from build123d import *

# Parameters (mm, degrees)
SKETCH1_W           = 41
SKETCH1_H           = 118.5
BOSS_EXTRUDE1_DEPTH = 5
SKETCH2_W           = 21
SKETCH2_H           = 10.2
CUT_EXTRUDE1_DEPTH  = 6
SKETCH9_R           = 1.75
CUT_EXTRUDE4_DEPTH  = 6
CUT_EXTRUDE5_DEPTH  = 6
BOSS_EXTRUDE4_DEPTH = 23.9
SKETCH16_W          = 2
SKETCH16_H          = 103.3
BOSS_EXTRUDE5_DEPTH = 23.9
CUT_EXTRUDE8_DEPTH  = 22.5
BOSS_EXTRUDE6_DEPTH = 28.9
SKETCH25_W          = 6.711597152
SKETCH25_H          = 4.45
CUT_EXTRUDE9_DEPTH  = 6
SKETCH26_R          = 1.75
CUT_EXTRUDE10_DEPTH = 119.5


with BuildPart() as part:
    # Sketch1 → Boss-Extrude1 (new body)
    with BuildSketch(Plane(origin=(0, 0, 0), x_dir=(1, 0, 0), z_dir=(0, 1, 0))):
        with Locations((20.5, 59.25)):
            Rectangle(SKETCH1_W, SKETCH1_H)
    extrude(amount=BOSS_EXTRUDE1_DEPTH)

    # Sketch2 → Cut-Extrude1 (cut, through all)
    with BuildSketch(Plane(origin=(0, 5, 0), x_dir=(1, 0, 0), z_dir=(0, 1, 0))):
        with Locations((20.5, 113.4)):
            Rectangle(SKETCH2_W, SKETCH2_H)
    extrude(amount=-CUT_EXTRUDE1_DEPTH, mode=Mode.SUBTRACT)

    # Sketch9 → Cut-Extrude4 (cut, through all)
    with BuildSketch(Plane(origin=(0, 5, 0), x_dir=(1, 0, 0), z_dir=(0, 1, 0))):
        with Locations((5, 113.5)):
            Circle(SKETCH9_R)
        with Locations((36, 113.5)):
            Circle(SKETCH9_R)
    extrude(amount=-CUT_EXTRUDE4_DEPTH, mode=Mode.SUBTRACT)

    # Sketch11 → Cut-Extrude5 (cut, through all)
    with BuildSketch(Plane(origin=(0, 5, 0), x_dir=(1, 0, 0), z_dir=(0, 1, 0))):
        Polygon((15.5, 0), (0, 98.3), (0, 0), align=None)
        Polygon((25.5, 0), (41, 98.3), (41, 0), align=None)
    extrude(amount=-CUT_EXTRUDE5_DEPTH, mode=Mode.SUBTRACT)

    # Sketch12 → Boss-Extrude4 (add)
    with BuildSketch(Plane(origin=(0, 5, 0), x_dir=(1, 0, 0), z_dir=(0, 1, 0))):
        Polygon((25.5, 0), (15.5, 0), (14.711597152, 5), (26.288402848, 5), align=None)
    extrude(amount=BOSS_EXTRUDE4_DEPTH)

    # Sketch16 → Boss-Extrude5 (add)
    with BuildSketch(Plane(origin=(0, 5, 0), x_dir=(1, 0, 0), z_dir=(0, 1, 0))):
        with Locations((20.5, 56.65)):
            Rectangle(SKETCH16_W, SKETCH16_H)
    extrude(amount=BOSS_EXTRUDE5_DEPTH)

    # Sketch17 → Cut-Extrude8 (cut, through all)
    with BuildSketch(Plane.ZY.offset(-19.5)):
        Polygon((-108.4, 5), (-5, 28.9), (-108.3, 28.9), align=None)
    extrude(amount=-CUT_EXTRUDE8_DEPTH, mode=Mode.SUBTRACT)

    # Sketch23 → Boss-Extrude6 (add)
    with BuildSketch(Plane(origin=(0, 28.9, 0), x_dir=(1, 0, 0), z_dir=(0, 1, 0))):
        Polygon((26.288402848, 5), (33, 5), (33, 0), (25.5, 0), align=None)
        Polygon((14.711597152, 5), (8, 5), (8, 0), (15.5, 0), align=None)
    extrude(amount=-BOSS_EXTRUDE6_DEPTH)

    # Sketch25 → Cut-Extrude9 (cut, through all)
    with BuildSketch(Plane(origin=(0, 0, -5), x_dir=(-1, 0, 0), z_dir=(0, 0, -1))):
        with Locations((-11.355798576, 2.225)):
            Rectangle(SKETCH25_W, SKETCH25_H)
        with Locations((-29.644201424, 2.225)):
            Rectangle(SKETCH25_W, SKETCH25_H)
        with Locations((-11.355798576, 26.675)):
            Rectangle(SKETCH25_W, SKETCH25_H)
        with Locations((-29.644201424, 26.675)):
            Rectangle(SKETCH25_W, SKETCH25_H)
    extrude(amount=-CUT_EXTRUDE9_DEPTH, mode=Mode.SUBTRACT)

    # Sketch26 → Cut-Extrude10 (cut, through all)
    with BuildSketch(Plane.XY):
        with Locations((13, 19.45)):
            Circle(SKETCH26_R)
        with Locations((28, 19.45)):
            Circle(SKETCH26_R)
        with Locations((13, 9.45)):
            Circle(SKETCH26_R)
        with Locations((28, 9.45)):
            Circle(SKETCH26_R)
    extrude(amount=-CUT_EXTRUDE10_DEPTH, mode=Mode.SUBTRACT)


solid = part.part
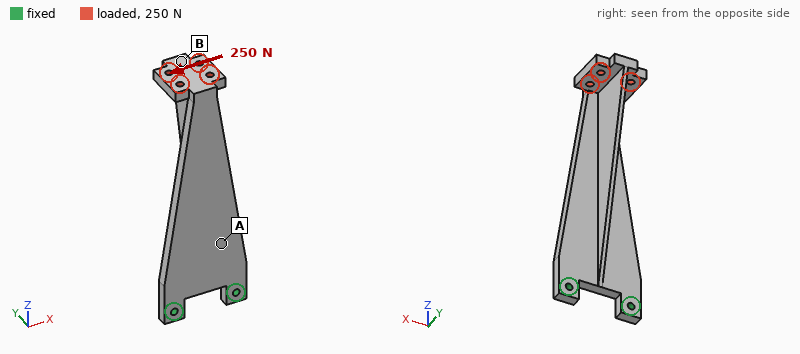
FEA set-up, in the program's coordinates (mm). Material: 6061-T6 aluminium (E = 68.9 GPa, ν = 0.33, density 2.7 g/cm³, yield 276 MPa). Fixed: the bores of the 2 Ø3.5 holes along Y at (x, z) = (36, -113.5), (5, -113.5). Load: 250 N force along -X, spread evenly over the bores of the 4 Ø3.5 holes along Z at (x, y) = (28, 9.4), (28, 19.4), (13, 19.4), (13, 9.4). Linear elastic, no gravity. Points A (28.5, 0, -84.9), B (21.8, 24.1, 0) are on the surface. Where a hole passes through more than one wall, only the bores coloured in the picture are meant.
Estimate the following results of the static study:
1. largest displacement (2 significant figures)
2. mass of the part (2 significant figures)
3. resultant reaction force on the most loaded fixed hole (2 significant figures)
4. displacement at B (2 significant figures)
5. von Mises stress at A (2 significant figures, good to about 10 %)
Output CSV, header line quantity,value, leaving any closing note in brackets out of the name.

quantity,value
largest displacement,0.45 mm
mass of the part,55 g
resultant reaction force on the most loaded fixed hole,870 N
displacement at B,0.39 mm
von Mises stress at A,18 MPa
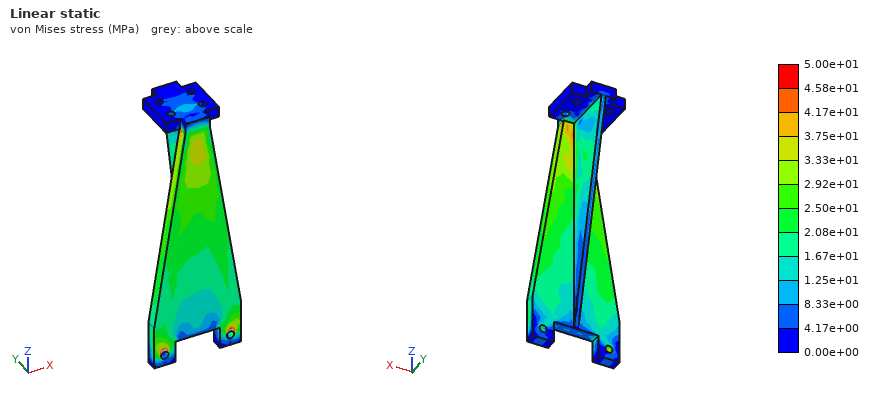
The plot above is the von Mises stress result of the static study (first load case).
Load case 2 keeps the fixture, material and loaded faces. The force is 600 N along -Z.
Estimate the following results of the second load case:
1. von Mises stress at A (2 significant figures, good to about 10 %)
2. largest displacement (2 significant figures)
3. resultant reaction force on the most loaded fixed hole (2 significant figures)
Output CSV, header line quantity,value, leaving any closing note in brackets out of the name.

quantity,value
von Mises stress at A,27 MPa
largest displacement,1.2 mm
resultant reaction force on the most loaded fixed hole,310 N
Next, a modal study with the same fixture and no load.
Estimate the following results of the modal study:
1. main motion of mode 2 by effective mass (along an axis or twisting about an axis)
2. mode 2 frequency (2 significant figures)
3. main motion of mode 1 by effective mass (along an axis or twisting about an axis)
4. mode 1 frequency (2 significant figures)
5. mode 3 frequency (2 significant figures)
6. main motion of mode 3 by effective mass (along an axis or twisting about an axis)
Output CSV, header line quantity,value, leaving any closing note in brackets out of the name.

quantity,value
main motion of mode 2 by effective mass,along X
mode 2 frequency,1300 Hz
main motion of mode 1 by effective mass,along Y
mode 1 frequency,310 Hz
mode 3 frequency,2800 Hz
main motion of mode 3 by effective mass,along Y
